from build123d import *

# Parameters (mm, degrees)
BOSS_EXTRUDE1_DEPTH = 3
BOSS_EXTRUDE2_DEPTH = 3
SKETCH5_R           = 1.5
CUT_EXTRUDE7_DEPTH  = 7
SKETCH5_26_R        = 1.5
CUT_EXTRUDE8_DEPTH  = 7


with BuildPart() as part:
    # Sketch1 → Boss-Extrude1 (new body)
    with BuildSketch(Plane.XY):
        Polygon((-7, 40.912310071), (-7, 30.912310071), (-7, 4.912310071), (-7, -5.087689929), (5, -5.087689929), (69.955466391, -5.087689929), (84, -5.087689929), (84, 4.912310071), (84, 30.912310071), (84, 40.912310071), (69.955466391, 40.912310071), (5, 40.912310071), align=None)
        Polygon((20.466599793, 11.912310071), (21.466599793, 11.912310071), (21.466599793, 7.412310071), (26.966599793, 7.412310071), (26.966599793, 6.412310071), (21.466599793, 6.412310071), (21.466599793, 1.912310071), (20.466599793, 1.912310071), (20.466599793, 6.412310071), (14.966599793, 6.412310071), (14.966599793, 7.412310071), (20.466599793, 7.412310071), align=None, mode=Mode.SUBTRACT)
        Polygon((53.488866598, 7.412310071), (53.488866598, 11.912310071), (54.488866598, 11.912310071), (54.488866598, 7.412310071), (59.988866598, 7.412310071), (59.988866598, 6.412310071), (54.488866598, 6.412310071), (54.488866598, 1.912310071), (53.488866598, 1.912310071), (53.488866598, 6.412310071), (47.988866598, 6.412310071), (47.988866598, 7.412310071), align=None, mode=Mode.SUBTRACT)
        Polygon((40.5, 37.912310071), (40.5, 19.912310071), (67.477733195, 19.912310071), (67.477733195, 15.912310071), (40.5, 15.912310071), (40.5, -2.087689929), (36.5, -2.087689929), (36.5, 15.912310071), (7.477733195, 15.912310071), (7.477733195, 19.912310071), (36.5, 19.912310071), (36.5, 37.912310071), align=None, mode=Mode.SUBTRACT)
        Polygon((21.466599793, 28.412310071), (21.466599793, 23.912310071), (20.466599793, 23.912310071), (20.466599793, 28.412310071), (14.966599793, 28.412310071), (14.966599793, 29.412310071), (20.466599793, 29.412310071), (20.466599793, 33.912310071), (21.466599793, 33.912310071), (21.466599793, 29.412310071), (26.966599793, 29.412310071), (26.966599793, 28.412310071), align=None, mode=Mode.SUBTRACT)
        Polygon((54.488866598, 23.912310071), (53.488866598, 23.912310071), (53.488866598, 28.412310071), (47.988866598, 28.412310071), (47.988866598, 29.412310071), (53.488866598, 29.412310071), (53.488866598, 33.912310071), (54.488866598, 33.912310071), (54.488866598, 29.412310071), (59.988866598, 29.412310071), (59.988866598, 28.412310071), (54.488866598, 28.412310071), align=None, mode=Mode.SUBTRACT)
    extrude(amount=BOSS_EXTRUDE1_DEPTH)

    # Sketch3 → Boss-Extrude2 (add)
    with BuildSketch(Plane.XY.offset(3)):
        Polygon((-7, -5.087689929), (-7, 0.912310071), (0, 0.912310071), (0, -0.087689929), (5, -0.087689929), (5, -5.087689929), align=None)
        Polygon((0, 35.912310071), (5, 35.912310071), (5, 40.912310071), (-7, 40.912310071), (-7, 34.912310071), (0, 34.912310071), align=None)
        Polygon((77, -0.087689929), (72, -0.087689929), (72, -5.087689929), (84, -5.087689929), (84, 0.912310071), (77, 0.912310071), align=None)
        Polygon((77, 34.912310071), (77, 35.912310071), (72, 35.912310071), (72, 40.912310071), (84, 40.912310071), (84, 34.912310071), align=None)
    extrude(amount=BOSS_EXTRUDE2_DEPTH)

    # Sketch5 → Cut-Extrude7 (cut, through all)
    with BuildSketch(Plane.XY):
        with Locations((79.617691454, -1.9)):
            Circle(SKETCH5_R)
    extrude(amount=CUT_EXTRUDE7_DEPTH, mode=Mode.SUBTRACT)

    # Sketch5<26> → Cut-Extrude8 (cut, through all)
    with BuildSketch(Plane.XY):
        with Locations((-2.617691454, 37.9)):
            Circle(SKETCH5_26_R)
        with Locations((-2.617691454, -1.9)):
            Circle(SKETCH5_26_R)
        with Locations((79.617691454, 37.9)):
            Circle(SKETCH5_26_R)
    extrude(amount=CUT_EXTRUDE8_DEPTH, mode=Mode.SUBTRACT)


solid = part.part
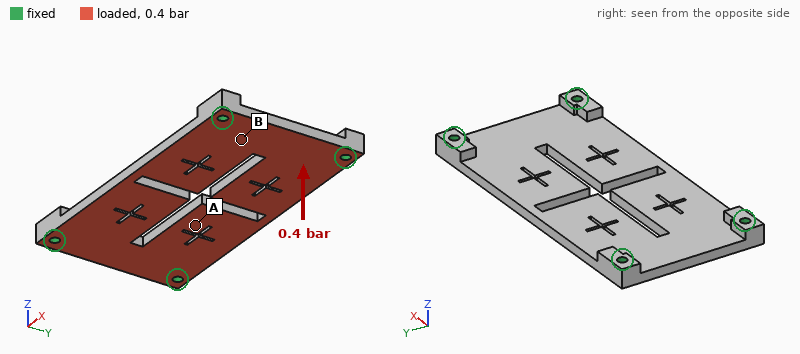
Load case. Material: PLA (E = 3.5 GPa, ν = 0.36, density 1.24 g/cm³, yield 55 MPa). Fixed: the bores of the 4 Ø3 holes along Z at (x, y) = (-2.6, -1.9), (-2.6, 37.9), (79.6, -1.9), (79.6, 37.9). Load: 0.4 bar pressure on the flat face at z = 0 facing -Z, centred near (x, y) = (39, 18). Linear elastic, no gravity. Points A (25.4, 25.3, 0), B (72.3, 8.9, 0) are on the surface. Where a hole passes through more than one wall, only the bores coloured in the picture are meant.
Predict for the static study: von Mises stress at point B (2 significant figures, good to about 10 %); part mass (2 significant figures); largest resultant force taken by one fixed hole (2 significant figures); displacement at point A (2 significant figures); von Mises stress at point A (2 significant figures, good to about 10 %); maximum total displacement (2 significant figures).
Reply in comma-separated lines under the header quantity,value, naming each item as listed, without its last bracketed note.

quantity,value
von Mises stress at point B,6.7 MPa
part mass,15 g
largest resultant force taken by one fixed hole,40 N
displacement at point A,0.64 mm
von Mises stress at point A,1.8 MPa
maximum total displacement,1.00 mm
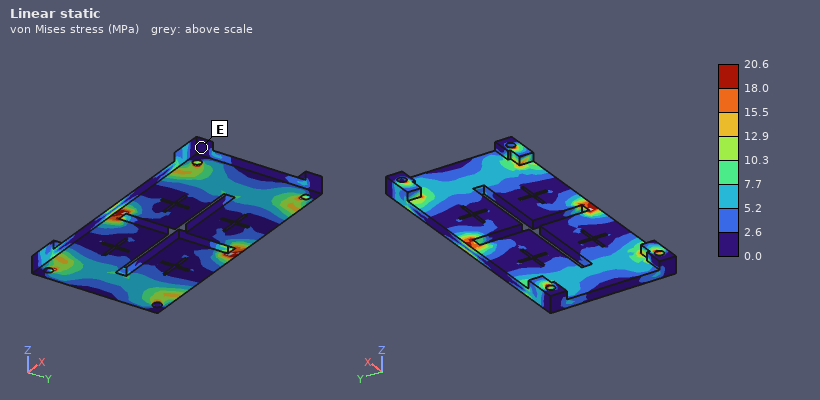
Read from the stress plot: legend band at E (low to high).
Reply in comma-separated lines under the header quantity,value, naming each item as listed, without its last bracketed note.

quantity,value
legend band at E,0.0 to 2.6 MPa
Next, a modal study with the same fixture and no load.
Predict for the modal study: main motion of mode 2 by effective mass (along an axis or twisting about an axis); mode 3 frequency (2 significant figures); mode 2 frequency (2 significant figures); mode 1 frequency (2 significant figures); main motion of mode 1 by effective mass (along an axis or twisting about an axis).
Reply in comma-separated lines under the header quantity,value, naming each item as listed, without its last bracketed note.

quantity,value
main motion of mode 2 by effective mass,twisting about X
mode 3 frequency,1300 Hz
mode 2 frequency,810 Hz
mode 1 frequency,690 Hz
main motion of mode 1 by effective mass,along Z
